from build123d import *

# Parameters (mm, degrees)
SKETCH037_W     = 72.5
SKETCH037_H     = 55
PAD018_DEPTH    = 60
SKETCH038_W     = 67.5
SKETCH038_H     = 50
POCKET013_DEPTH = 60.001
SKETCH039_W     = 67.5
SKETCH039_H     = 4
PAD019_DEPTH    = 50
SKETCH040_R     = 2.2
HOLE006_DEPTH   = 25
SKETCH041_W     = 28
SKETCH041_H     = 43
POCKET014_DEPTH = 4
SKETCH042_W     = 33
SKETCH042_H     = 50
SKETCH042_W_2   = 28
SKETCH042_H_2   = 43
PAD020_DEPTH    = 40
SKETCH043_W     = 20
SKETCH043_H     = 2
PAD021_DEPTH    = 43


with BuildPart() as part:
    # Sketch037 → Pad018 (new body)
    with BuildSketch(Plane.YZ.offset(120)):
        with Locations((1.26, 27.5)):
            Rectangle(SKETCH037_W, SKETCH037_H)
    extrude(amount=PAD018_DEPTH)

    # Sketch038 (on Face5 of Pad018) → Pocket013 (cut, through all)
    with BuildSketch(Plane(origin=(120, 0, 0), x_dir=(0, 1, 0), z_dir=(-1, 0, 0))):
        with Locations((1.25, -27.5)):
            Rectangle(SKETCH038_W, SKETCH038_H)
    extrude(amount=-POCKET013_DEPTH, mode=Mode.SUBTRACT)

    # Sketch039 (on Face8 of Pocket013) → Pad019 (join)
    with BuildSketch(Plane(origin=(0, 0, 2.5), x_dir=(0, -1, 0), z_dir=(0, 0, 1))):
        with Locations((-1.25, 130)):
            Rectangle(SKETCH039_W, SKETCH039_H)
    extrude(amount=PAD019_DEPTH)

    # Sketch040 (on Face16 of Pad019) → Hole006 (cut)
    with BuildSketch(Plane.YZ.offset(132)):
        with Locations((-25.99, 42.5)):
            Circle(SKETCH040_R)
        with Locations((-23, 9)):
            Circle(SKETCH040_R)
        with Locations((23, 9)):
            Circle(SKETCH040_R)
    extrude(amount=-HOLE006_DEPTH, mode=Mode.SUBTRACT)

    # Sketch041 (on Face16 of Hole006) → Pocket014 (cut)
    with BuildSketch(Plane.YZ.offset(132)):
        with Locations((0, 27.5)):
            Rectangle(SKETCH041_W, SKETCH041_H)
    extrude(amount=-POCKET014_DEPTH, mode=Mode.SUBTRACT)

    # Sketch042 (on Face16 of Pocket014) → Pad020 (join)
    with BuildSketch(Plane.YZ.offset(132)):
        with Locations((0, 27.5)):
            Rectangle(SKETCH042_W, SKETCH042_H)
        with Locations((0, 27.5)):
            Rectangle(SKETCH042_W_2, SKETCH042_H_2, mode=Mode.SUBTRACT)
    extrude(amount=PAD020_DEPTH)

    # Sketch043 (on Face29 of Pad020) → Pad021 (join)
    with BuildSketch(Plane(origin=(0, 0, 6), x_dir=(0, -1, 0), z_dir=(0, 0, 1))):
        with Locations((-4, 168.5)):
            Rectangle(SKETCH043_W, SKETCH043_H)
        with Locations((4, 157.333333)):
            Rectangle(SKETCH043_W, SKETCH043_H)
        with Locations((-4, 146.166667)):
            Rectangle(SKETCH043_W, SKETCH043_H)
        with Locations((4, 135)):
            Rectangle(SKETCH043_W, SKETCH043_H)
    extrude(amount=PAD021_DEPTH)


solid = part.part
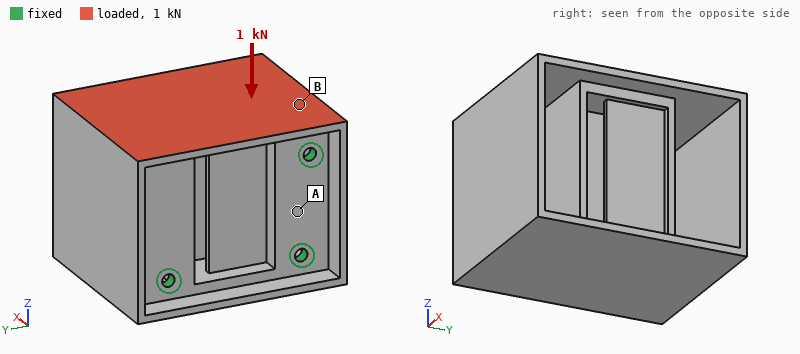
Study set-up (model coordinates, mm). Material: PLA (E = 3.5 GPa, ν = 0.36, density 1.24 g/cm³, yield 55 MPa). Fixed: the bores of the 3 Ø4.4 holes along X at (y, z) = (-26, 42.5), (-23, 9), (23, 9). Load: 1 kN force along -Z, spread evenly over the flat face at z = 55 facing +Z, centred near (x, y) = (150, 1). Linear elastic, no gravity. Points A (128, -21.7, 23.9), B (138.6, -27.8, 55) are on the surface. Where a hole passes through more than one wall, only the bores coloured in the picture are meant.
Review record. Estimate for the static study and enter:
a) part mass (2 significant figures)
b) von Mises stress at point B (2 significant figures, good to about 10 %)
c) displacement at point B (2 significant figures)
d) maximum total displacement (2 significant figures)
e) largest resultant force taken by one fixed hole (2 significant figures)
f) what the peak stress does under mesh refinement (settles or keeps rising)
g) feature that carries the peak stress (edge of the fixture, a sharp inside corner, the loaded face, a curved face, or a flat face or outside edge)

87 g
4.0 MPa
0.15 mm
0.74 mm
640 N
keeps rising
edge of the fixture
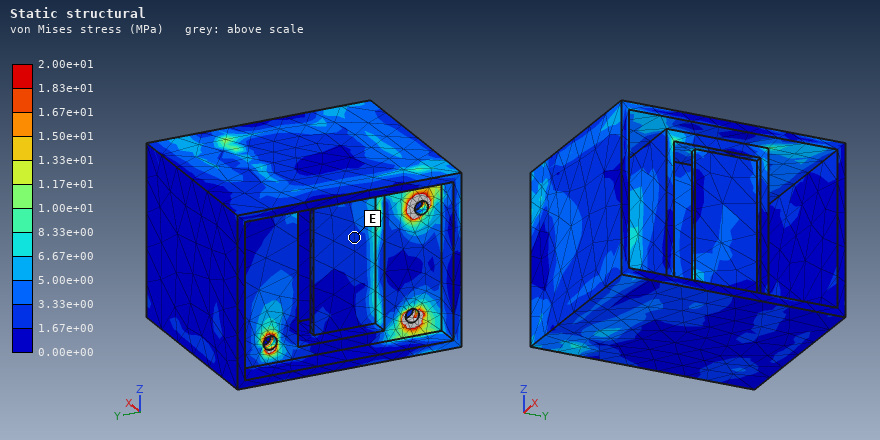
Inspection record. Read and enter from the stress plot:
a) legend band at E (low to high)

1.67e+00 to 3.33e+00 MPa
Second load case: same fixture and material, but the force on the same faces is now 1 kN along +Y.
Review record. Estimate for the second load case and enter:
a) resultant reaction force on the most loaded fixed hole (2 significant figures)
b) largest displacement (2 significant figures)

710 N
0.65 mm
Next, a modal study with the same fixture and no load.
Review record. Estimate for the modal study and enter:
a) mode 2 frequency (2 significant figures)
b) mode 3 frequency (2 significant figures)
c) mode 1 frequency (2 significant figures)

1300 Hz
1500 Hz
710 Hz
